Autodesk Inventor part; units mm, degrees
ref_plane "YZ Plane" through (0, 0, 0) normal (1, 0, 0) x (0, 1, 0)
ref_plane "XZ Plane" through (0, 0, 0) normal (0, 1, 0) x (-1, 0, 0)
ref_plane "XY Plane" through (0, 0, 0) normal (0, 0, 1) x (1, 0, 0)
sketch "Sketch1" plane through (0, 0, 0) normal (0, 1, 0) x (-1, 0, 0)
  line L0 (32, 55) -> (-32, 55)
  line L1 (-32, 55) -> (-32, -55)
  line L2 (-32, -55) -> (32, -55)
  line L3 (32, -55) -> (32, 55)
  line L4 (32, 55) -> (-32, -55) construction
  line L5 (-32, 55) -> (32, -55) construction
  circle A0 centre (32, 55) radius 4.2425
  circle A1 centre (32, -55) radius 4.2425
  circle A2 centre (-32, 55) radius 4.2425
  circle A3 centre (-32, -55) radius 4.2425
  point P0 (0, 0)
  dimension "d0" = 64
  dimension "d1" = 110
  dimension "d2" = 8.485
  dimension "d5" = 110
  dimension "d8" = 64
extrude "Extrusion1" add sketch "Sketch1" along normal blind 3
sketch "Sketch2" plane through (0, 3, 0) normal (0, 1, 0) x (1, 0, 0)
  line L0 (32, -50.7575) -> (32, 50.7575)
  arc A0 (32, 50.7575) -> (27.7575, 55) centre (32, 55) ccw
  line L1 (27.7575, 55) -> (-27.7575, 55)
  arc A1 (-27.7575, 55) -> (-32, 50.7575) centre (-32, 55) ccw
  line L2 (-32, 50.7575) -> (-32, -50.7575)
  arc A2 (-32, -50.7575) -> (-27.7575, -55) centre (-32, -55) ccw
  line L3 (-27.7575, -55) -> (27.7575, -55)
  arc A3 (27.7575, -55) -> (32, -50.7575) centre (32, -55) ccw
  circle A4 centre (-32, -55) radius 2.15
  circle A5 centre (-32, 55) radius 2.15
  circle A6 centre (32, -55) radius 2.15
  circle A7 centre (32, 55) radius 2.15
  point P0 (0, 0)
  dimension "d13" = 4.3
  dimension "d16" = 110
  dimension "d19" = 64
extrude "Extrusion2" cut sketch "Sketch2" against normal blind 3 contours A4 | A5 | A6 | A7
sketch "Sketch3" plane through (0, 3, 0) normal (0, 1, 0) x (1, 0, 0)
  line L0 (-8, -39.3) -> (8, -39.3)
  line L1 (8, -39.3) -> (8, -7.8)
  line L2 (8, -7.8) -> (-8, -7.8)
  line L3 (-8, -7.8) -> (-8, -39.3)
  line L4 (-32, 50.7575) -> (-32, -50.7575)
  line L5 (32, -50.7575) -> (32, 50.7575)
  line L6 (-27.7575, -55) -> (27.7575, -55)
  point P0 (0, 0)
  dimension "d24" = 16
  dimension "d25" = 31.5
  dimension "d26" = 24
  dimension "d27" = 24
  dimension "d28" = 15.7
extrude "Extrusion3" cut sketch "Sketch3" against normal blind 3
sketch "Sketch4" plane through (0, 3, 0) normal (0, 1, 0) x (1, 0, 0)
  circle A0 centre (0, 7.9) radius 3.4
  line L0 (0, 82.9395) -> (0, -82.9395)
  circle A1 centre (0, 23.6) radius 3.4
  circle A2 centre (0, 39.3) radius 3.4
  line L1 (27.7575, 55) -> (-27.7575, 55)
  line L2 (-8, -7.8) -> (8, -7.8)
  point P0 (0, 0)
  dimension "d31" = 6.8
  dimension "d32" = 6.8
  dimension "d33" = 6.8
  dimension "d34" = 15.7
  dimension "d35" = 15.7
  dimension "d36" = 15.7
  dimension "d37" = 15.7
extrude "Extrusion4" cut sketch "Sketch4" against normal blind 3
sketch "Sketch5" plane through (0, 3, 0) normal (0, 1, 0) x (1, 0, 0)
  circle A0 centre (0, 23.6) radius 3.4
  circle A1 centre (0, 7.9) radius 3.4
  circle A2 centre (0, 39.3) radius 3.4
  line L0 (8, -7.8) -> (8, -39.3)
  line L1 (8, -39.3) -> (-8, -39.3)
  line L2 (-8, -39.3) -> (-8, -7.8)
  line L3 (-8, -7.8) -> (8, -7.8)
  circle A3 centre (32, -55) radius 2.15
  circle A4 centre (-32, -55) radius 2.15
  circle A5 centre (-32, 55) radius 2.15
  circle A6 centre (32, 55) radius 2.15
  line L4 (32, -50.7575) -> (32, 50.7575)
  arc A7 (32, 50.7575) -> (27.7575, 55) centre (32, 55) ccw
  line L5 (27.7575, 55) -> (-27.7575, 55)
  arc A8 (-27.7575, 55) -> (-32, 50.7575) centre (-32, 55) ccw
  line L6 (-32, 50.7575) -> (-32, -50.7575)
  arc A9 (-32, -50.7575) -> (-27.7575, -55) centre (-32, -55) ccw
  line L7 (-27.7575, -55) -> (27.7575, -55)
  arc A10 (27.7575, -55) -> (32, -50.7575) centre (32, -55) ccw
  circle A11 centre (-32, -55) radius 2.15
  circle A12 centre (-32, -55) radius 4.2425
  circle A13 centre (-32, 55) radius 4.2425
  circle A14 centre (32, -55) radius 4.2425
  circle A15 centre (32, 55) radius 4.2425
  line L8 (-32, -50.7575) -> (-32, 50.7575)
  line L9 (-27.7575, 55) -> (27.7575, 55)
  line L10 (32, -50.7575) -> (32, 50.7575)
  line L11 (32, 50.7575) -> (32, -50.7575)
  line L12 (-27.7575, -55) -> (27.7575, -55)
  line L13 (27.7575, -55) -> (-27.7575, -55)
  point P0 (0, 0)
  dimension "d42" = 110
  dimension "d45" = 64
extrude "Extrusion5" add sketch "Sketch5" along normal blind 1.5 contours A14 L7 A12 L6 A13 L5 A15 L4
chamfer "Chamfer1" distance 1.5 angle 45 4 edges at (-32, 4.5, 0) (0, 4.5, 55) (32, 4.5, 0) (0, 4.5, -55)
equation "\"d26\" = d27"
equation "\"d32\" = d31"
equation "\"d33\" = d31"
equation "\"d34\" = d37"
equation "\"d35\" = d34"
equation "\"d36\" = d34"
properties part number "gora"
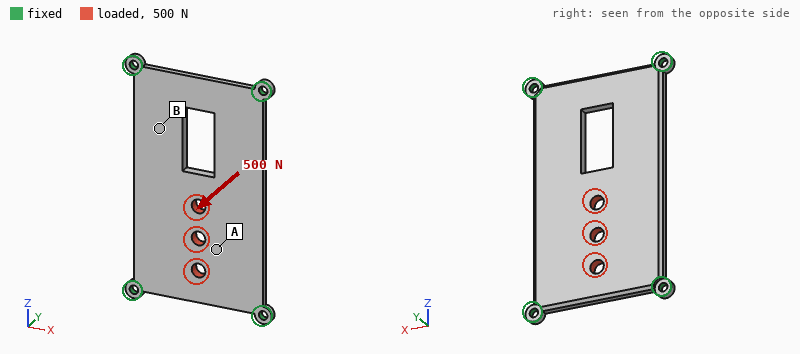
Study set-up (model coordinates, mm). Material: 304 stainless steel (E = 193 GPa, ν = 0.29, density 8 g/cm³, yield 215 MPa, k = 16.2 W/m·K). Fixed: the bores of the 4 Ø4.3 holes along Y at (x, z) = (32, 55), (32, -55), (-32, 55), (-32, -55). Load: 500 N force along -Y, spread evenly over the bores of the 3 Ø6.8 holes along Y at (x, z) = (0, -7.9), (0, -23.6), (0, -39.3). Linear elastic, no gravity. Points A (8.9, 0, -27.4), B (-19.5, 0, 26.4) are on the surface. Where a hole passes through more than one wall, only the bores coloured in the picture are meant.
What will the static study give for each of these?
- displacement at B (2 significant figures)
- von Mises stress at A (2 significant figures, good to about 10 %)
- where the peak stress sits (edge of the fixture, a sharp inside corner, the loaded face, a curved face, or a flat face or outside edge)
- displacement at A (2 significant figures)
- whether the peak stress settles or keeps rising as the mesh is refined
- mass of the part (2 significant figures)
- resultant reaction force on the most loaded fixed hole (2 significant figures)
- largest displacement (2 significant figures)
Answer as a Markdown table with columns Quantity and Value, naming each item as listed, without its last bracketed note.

| Quantity | Value |
|---|---|
| displacement at B | 37 µm |
| von Mises stress at A | 20 MPa |
| where the peak stress sits | edge of the fixture |
| displacement at A | 54 µm |
| whether the peak stress settles or keeps rising as the mesh is refined | keeps rising |
| mass of the part | 230 g |
| resultant reaction force on the most loaded fixed hole | 330 N |
| largest displacement | 68 µm |
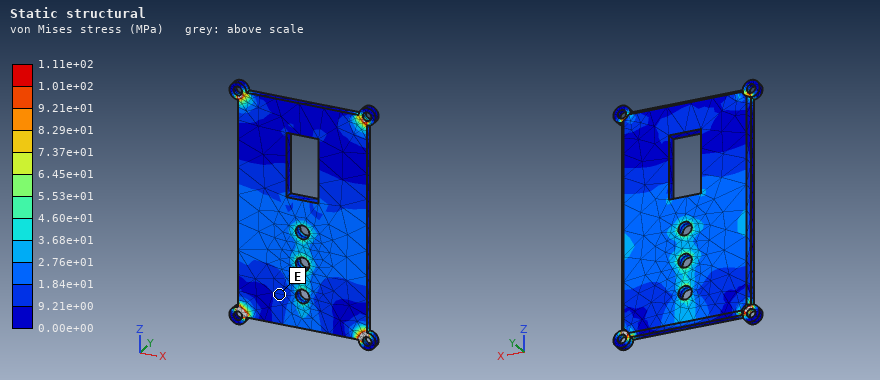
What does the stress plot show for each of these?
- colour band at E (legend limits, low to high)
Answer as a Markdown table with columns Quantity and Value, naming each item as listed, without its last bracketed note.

| Quantity | Value |
|---|---|
| colour band at E | 9.21e+00 to 1.84e+01 MPa |
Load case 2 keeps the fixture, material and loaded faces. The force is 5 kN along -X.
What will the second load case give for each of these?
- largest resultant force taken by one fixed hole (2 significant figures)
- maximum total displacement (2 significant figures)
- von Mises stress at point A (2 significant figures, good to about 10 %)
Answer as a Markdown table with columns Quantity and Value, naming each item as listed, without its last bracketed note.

| Quantity | Value |
|---|---|
| largest resultant force taken by one fixed hole | 2.3 kN |
| maximum total displacement | 12 µm |
| von Mises stress at point A | 18 MPa |
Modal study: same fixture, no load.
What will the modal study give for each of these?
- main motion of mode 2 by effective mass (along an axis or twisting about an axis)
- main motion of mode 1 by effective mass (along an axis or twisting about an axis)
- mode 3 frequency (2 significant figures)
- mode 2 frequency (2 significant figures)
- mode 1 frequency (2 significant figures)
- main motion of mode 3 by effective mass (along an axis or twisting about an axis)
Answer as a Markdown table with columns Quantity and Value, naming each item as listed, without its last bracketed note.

| Quantity | Value |
|---|---|
| main motion of mode 2 by effective mass | twisting about Z |
| main motion of mode 1 by effective mass | along Y |
| mode 3 frequency | 3300 Hz |
| mode 2 frequency | 2400 Hz |
| mode 1 frequency | 1200 Hz |
| main motion of mode 3 by effective mass | twisting about X |
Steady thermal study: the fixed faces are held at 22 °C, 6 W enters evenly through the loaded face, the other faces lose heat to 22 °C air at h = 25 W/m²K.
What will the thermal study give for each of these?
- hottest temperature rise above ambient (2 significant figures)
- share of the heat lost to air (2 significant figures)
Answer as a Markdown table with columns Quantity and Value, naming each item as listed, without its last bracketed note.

| Quantity | Value |
|---|---|
| hottest temperature rise above ambient | 28 K |
| share of the heat lost to air | 72 % |
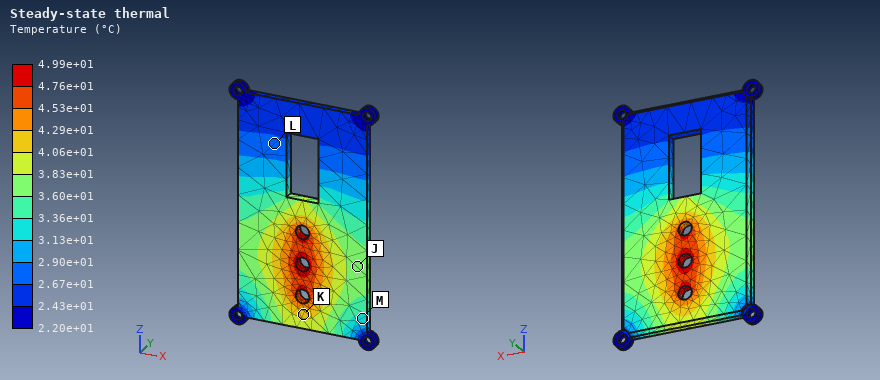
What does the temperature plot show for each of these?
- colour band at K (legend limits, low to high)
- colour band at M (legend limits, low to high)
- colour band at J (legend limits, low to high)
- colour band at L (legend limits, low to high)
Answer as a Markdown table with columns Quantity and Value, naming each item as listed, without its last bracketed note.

| Quantity | Value |
|---|---|
| colour band at K | 4.06e+01 to 4.29e+01 °C |
| colour band at M | 3.13e+01 to 3.36e+01 °C |
| colour band at J | 3.60e+01 to 3.83e+01 °C |
| colour band at L | 2.67e+01 to 2.90e+01 °C |
